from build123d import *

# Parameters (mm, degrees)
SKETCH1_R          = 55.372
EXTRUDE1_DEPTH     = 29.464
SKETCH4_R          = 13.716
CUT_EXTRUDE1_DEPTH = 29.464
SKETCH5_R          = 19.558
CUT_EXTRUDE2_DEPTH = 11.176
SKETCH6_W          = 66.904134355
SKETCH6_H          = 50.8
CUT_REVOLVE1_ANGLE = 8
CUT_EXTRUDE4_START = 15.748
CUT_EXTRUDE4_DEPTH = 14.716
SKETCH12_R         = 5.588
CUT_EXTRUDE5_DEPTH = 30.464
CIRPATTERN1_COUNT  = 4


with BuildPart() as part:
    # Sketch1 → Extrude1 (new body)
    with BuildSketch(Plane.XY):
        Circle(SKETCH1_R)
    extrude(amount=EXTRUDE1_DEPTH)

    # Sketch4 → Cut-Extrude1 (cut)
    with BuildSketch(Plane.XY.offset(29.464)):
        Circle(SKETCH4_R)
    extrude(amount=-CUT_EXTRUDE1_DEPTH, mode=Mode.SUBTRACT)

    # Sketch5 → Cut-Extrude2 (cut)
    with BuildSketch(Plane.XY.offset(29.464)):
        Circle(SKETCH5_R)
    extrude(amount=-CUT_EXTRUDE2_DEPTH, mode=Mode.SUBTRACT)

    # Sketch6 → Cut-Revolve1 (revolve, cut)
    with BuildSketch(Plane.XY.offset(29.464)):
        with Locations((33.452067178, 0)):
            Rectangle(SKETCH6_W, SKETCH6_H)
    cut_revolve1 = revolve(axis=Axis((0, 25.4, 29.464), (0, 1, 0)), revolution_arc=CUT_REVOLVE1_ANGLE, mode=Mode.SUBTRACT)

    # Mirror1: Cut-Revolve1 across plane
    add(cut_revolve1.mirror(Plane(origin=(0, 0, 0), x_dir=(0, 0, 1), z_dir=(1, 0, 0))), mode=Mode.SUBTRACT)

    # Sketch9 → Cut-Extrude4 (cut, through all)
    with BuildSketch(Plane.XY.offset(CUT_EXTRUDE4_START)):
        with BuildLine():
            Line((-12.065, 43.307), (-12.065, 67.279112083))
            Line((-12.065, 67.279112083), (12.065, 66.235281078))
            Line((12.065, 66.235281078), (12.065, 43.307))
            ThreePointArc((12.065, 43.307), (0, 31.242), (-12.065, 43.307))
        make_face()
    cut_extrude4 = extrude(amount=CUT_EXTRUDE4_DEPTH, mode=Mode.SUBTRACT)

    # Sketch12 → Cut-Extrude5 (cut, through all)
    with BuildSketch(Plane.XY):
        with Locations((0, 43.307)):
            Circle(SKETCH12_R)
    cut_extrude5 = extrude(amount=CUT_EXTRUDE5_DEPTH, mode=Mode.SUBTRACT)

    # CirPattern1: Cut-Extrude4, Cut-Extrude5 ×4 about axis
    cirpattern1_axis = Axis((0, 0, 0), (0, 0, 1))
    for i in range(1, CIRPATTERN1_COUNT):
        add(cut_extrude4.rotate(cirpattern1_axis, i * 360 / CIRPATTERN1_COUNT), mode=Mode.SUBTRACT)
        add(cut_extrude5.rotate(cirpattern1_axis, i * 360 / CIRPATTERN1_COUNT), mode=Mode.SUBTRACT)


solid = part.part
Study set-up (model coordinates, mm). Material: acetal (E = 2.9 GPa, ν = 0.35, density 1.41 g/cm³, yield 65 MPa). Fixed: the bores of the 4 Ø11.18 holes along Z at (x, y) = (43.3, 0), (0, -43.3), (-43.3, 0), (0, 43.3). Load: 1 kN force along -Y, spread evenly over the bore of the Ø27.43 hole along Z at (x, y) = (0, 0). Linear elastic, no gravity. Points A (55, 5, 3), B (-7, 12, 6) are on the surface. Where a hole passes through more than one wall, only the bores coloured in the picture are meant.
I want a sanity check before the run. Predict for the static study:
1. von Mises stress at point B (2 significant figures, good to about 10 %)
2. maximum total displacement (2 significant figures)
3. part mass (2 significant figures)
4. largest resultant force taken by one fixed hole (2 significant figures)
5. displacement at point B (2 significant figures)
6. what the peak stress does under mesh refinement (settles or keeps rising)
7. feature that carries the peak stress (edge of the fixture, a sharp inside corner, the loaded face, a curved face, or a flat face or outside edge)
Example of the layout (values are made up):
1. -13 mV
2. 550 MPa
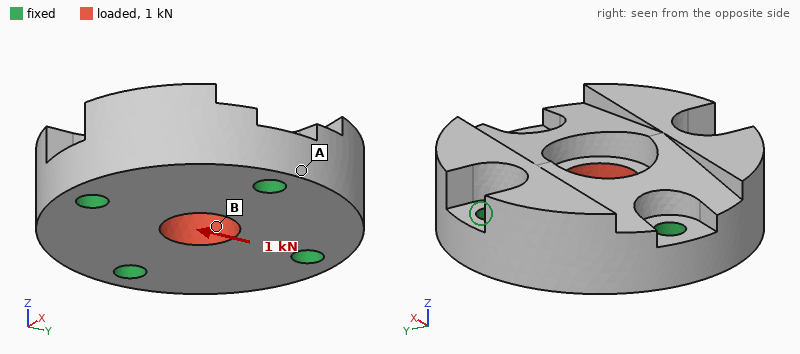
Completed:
1. 0.76 MPa
2. 7.9 µm
3. 300 g
4. 320 N
5. 7.2 µm
6. keeps rising
7. edge of the fixture
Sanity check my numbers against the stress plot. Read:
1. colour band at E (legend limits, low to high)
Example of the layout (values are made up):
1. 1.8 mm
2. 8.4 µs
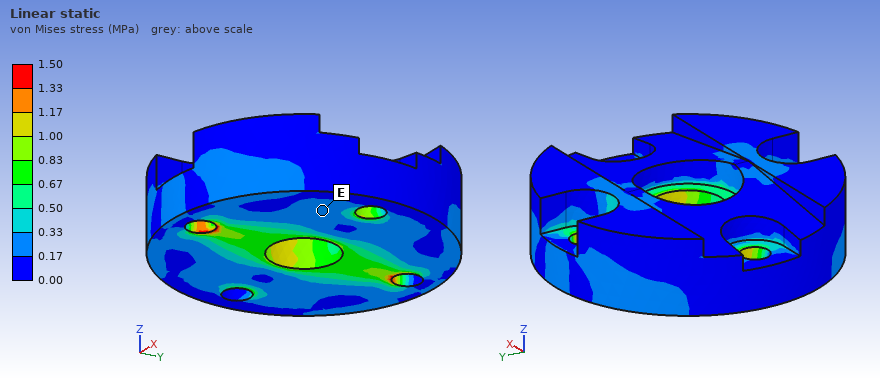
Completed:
1. 0.17 to 0.33 MPa
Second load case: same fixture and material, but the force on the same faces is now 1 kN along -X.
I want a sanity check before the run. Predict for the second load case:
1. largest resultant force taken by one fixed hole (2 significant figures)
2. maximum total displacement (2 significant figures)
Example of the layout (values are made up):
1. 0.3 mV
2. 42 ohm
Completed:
1. 320 N
2. 7.9 µm
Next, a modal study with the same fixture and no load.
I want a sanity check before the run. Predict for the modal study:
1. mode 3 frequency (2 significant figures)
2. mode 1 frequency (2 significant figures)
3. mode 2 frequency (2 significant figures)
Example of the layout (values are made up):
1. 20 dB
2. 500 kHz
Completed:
1. 3700 Hz
2. 3400 Hz
3. 3600 Hz
